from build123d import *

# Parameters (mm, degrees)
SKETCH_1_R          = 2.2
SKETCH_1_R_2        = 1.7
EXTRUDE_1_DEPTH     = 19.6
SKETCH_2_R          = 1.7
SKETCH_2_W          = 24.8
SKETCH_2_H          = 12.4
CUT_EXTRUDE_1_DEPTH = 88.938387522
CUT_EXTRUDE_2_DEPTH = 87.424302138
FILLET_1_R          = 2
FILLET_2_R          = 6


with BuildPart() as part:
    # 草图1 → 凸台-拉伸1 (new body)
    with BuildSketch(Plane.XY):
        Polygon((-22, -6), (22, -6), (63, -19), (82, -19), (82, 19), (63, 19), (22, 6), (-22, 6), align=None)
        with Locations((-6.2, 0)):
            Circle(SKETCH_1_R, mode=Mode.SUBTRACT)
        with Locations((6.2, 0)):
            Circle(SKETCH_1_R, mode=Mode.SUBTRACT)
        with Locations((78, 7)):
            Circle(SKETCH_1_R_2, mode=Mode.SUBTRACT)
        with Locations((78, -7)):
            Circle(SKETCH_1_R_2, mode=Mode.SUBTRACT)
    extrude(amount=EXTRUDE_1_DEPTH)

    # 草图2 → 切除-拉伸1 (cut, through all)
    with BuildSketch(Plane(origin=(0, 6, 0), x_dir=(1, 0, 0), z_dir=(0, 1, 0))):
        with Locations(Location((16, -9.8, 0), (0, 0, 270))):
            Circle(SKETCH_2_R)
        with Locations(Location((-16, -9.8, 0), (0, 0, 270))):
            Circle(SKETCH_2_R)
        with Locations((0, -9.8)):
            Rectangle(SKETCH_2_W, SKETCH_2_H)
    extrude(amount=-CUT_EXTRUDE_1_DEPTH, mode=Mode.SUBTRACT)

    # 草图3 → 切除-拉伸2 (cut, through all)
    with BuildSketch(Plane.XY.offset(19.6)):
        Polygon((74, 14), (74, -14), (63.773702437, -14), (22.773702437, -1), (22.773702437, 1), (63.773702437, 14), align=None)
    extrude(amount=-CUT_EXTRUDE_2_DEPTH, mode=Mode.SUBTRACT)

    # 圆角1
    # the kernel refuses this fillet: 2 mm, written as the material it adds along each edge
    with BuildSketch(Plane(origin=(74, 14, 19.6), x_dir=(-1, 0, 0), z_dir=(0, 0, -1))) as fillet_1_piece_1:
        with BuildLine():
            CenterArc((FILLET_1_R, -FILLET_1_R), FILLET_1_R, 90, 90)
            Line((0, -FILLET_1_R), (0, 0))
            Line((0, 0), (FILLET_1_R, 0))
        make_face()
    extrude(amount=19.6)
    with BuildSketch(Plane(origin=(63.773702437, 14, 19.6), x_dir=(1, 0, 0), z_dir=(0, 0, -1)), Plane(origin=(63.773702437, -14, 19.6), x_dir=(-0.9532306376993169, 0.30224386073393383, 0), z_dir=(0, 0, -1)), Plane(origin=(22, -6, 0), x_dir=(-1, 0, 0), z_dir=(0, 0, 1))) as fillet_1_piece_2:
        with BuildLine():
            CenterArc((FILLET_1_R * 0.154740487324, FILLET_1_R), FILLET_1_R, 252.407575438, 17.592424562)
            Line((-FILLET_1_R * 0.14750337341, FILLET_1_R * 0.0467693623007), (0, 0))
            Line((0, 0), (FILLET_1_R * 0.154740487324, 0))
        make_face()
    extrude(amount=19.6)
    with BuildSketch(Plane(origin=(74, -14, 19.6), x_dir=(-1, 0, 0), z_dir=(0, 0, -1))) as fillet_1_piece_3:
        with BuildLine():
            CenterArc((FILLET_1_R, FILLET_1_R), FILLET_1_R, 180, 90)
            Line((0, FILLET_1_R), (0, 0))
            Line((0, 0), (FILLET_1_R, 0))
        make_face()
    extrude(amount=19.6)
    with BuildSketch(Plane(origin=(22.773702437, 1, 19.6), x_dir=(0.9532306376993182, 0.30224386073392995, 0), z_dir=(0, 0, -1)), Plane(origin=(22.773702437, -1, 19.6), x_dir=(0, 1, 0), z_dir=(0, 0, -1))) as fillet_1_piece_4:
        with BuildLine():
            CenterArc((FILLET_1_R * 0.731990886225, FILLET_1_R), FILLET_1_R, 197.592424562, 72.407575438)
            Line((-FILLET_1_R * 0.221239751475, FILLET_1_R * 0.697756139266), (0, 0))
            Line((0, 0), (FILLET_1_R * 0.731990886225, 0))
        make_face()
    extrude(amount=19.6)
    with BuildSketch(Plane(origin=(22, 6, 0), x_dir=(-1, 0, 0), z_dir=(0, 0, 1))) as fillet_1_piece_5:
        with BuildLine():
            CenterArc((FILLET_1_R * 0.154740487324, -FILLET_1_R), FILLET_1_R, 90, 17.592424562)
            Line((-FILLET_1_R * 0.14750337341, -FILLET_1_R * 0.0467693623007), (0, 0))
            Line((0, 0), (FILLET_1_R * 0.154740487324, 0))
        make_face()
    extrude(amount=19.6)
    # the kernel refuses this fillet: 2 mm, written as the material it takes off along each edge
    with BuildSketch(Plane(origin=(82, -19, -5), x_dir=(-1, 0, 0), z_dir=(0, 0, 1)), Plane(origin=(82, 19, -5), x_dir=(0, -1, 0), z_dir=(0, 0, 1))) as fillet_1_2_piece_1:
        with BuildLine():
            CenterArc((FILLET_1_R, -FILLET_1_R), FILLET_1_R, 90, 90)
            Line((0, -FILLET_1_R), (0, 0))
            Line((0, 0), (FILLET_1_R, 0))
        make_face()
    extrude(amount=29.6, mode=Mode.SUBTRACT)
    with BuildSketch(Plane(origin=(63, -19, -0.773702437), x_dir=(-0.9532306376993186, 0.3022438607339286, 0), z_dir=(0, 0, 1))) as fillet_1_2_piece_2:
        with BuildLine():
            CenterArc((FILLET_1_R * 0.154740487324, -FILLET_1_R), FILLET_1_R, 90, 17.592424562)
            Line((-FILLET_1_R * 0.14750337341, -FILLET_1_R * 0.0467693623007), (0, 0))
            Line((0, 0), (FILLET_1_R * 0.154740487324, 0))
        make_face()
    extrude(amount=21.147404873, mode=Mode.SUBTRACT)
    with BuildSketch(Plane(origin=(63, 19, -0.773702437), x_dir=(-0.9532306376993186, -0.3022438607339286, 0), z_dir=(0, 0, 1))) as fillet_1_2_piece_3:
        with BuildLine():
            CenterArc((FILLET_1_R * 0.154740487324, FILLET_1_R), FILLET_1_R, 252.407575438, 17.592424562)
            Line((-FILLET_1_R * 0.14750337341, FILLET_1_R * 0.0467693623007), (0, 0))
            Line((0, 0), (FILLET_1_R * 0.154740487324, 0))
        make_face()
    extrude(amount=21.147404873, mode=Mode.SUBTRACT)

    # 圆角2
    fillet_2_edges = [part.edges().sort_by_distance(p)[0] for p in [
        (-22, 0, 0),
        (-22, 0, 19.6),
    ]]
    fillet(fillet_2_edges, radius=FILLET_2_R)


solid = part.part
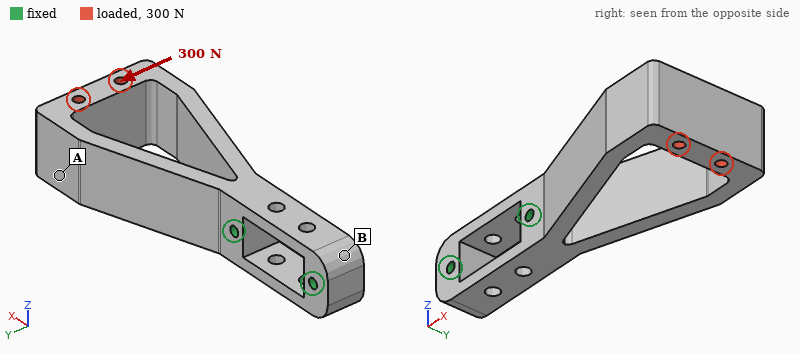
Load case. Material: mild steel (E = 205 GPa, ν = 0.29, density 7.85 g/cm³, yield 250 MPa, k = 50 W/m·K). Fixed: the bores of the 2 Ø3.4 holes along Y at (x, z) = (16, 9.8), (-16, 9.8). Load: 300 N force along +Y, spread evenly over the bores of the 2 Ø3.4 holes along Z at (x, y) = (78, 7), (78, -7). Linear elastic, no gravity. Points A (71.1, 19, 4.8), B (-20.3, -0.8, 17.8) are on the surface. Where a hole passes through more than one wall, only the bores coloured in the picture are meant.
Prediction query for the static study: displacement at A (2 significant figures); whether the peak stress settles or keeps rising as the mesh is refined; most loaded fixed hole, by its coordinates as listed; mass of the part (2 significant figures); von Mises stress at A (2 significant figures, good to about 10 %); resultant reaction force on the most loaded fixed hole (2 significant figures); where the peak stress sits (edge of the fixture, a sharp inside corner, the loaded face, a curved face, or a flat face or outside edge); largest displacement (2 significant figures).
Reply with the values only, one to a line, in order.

0.14 mm
keeps rising
(16, 9.8)
170 g
33 MPa
410 N
edge of the fixture
0.16 mm
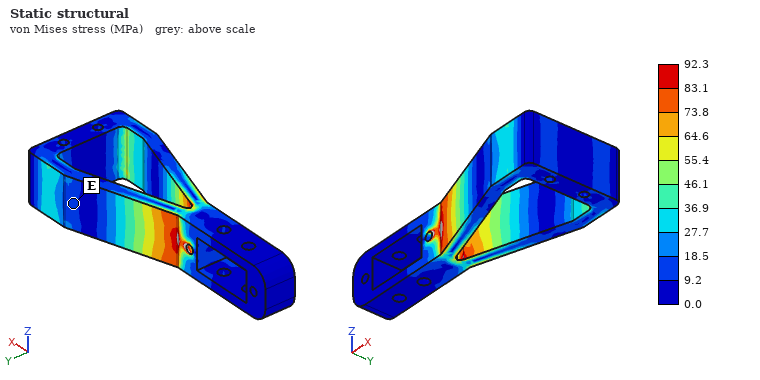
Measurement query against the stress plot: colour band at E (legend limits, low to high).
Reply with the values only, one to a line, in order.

9.2 to 18.5 MPa
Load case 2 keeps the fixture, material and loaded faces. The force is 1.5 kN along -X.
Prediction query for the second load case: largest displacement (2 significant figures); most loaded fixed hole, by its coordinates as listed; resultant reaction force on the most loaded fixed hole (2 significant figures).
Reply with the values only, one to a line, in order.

11 µm
(16, 9.8)
1.4 kN
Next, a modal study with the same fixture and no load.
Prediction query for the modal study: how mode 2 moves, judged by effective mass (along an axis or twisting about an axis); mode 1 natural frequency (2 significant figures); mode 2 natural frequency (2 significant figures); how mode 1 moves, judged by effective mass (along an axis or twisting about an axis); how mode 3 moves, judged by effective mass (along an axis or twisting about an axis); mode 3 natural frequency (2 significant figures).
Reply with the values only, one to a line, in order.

along Z
870 Hz
1700 Hz
along Y
twisting about X
3700 Hz
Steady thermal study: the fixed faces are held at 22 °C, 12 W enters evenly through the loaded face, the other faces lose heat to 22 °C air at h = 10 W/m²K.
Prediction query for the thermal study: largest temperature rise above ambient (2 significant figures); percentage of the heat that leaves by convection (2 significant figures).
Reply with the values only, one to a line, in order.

68 K
26 %
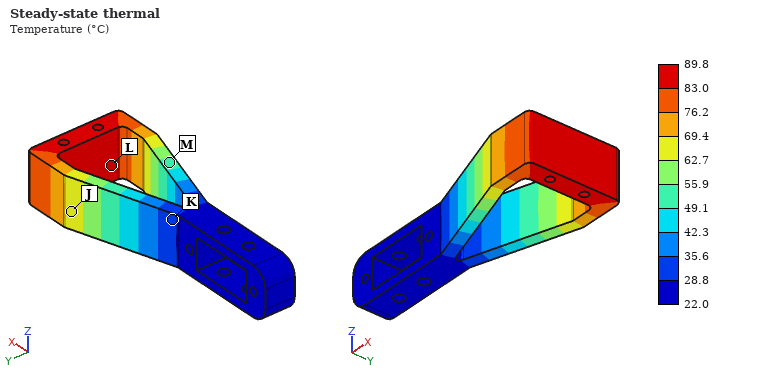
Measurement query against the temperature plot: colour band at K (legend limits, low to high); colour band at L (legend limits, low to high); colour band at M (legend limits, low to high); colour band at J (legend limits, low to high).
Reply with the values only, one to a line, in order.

28.8 to 35.6 °C
83.0 to 89.8 °C
49.1 to 55.9 °C
62.7 to 69.4 °C
